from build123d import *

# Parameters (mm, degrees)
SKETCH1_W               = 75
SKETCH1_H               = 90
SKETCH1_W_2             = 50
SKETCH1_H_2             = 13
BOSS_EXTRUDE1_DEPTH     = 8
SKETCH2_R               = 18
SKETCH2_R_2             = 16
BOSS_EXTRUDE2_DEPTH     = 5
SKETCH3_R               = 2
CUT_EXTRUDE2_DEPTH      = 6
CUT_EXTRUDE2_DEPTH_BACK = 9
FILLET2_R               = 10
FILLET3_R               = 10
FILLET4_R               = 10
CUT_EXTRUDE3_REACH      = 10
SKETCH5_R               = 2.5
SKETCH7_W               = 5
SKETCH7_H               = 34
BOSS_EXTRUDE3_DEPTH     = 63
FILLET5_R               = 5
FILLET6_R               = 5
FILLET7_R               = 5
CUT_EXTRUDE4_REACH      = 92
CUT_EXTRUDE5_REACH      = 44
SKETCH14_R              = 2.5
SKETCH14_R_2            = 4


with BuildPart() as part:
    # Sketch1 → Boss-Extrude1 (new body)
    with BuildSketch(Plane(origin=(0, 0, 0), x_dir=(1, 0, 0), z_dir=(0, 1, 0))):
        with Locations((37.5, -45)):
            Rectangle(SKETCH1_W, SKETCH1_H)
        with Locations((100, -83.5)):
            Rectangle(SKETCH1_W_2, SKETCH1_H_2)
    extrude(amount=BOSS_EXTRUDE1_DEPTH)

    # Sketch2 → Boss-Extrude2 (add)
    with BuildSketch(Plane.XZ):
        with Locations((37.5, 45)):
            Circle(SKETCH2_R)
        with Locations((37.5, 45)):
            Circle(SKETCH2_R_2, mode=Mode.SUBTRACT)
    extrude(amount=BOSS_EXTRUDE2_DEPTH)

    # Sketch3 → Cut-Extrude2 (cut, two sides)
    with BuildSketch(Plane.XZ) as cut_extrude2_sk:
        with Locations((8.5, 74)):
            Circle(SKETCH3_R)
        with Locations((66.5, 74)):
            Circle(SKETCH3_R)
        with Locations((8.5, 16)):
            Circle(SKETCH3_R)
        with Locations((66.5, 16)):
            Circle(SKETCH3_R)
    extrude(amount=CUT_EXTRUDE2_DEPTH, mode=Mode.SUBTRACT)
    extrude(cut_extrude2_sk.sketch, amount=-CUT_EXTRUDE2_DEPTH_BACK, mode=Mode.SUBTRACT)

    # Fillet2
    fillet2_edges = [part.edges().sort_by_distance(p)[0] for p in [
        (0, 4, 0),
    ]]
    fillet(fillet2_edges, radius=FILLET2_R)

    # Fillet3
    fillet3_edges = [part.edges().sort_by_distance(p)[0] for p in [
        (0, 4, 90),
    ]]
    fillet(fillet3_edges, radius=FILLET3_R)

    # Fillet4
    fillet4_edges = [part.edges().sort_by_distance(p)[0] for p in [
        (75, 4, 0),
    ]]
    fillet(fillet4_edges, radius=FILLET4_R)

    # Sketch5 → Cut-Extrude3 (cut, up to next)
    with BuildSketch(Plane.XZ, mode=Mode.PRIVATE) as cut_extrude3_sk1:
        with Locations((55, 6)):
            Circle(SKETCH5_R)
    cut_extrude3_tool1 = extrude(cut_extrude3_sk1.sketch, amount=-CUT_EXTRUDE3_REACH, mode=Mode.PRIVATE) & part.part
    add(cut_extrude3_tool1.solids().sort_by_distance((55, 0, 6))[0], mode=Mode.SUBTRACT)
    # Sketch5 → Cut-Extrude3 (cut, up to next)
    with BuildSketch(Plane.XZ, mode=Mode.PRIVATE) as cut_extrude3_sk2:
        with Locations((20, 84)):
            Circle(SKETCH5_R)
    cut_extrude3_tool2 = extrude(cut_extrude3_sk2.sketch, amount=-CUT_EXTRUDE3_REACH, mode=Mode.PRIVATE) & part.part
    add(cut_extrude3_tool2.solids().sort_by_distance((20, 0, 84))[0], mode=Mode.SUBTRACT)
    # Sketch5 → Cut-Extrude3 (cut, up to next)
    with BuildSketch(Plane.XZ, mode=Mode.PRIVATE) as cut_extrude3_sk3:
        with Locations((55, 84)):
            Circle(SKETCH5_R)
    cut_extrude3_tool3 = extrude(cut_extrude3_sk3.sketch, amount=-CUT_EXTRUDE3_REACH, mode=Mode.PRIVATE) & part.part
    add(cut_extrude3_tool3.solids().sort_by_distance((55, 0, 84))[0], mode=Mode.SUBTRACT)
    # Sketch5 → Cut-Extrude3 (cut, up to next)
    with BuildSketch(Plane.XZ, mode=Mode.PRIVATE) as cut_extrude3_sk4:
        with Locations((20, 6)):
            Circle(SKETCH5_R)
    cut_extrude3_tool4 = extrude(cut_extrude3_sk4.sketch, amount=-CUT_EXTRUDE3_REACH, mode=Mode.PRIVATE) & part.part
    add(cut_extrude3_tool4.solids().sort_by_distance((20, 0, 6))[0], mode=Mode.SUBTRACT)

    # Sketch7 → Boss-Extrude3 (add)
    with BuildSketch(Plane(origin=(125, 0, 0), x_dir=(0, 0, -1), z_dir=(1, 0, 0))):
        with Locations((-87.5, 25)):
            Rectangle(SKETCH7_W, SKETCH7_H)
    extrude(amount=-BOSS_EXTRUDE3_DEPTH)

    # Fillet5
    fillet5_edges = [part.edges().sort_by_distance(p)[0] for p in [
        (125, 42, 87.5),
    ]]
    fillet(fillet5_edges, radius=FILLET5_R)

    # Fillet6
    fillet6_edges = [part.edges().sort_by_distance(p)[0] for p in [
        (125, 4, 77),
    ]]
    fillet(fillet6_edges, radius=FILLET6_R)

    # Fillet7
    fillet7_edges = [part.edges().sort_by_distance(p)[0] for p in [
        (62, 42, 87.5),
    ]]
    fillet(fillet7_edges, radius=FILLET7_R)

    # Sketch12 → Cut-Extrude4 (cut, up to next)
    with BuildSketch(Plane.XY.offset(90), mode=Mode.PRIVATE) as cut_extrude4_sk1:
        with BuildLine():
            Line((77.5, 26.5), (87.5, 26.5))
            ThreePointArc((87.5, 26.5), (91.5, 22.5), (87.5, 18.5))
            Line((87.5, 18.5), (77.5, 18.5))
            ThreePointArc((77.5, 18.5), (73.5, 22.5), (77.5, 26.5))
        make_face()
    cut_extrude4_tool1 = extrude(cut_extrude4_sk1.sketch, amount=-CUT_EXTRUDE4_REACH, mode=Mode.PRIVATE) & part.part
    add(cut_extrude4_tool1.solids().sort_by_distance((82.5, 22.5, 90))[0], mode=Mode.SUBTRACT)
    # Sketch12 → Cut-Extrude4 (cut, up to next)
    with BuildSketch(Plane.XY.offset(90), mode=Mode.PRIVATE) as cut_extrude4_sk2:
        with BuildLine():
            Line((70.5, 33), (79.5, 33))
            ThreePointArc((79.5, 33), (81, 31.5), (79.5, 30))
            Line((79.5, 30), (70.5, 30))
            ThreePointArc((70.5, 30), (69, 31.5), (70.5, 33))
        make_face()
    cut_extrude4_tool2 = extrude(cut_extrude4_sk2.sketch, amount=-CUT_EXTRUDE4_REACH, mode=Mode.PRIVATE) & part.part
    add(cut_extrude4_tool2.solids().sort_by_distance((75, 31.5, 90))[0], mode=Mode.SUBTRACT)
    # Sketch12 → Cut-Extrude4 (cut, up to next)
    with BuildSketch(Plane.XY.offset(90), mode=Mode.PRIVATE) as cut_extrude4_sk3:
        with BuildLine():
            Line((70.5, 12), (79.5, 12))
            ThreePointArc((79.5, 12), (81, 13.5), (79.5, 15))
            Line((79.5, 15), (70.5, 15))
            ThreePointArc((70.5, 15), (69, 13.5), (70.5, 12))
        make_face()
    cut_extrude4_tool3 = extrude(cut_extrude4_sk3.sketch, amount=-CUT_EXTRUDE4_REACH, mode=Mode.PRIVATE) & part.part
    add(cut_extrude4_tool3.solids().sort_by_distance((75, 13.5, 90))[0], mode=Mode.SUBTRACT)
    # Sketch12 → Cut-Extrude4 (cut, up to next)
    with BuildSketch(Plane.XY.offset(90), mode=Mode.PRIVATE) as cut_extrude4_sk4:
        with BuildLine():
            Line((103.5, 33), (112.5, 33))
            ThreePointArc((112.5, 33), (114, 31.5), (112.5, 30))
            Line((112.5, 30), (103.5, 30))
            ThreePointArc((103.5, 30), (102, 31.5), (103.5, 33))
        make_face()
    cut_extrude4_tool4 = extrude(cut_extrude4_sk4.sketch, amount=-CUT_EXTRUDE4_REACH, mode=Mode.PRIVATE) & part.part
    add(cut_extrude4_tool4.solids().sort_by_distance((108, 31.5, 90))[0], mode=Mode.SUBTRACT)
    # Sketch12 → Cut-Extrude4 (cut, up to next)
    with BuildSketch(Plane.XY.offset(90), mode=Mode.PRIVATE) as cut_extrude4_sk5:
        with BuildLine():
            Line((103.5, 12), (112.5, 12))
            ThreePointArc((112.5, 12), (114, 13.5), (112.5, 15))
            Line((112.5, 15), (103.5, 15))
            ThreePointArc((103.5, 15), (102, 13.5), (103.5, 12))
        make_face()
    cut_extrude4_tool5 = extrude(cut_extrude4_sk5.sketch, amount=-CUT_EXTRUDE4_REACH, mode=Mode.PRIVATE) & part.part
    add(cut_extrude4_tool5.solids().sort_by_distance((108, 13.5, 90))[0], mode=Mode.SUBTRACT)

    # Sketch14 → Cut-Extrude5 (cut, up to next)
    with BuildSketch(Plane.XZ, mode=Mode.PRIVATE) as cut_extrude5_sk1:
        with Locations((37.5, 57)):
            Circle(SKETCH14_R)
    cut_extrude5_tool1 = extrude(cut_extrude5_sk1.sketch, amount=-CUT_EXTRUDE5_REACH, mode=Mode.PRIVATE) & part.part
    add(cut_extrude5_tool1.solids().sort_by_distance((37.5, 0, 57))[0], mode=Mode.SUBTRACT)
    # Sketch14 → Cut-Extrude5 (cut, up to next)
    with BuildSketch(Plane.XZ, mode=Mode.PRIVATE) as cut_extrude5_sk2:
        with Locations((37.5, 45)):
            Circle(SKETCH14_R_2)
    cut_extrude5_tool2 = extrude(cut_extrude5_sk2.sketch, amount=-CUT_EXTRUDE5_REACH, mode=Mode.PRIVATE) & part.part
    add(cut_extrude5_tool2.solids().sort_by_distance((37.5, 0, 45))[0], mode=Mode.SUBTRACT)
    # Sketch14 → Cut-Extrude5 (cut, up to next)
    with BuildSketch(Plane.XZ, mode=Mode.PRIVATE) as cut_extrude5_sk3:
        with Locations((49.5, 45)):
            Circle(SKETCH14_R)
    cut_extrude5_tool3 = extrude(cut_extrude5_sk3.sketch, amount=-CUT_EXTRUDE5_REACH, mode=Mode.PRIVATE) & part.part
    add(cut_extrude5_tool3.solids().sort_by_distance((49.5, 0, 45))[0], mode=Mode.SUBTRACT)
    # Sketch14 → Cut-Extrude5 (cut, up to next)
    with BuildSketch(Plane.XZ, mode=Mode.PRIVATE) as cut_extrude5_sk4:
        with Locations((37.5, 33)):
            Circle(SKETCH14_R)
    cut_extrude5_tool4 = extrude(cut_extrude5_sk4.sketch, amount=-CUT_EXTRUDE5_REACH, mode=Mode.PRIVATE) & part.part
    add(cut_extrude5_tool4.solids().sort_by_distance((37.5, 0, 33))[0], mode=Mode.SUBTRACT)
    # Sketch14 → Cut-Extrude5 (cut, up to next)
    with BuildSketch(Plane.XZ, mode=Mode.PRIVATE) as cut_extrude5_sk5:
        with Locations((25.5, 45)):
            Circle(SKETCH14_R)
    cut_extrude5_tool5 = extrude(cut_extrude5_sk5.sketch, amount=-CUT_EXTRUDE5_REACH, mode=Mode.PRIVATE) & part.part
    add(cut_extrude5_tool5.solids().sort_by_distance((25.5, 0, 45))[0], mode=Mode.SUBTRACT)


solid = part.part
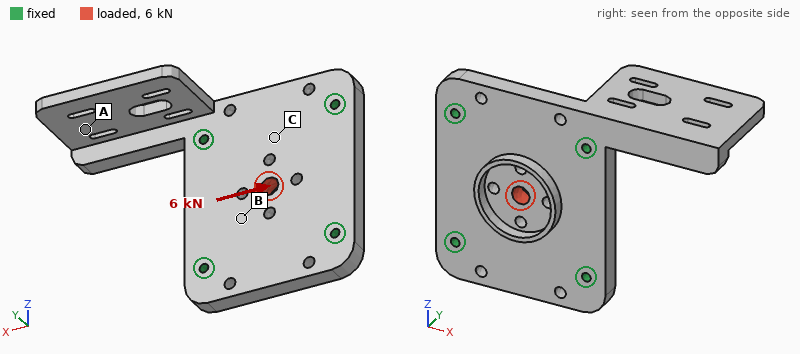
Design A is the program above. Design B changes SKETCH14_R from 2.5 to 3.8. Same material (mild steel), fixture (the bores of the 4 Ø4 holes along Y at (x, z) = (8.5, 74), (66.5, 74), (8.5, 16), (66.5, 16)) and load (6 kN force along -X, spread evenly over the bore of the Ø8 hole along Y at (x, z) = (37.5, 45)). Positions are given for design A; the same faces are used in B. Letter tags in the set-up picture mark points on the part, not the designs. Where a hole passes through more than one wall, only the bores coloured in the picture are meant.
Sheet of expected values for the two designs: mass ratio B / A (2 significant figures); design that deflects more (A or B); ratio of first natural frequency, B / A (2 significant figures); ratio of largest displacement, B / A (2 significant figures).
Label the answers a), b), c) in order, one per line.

a) 0.99
b) B
c) 1.0
d) 1.2
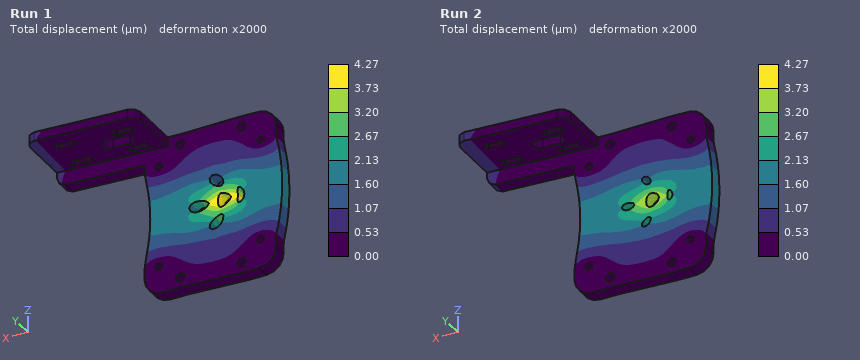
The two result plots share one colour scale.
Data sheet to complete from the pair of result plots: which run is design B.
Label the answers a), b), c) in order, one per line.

a) Run 1
